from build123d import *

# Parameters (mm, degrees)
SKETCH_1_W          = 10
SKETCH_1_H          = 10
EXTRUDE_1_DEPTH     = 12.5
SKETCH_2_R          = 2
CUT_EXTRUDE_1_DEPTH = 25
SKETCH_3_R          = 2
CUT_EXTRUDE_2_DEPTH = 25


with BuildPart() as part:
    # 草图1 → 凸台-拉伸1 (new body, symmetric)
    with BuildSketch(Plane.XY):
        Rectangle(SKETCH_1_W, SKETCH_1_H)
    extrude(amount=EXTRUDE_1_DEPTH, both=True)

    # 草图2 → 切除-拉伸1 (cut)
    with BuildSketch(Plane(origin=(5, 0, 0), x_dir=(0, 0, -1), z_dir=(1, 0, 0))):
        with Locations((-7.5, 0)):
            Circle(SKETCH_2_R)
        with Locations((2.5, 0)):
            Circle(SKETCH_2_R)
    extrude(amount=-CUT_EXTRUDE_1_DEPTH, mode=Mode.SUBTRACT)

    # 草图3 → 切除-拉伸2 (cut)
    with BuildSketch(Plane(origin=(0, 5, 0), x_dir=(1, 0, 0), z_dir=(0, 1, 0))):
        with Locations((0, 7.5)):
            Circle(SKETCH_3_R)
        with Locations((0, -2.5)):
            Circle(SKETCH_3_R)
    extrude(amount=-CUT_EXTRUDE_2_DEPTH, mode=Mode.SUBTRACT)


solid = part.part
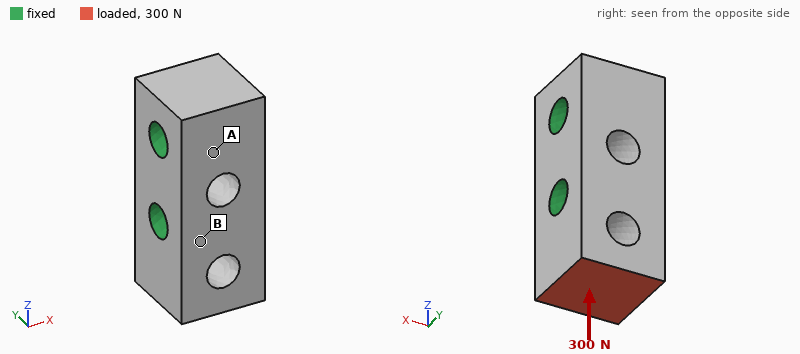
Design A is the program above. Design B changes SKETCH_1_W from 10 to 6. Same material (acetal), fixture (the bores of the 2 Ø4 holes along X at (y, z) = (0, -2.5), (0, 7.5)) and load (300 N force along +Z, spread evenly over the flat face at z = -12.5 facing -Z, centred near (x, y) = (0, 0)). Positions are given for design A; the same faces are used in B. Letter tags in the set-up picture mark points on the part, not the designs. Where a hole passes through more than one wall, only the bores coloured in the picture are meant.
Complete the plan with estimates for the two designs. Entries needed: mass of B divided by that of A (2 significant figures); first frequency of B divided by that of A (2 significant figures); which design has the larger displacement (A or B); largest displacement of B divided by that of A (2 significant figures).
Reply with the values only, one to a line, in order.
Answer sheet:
0.55
0.70
B
2.2
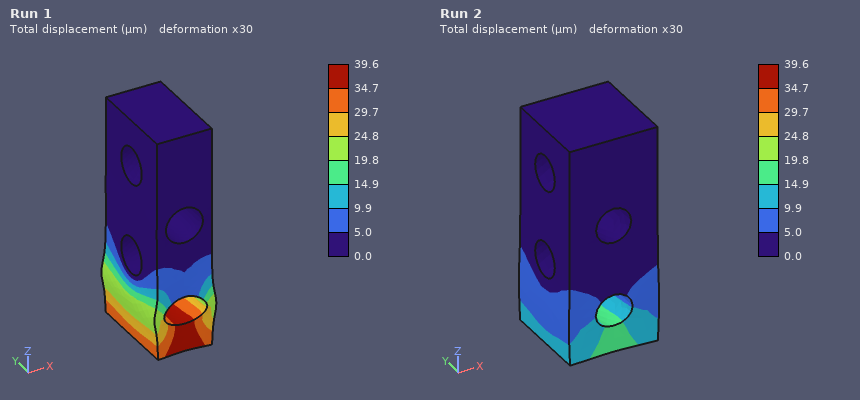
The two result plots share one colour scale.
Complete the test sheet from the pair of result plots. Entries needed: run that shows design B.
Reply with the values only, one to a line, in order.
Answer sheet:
Run 1
